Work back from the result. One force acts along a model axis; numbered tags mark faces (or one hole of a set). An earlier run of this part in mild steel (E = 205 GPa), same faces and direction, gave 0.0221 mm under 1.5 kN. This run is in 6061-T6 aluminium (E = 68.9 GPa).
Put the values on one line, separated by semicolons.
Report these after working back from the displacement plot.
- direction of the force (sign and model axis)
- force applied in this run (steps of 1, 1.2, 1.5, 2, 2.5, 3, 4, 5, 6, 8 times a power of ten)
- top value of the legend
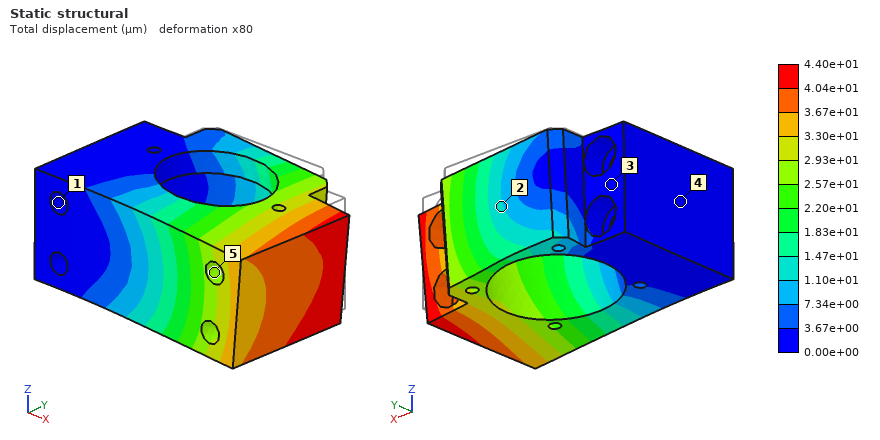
-Z; 1 kN; 4.40e+01 µm
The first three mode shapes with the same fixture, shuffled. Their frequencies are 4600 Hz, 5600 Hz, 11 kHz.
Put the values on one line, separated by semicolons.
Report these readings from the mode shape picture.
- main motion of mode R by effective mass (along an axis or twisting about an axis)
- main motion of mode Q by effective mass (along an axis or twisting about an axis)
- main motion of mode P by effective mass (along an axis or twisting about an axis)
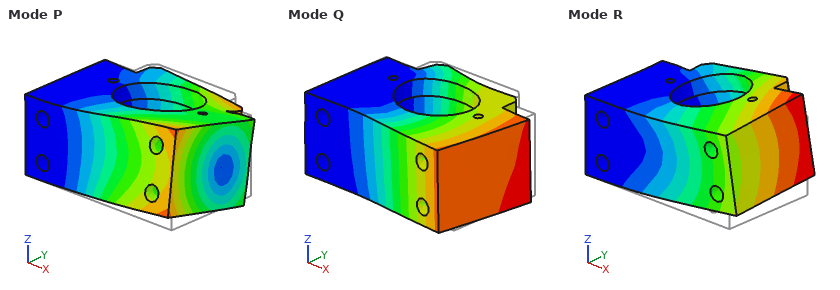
along Z; along Y; twisting about X
